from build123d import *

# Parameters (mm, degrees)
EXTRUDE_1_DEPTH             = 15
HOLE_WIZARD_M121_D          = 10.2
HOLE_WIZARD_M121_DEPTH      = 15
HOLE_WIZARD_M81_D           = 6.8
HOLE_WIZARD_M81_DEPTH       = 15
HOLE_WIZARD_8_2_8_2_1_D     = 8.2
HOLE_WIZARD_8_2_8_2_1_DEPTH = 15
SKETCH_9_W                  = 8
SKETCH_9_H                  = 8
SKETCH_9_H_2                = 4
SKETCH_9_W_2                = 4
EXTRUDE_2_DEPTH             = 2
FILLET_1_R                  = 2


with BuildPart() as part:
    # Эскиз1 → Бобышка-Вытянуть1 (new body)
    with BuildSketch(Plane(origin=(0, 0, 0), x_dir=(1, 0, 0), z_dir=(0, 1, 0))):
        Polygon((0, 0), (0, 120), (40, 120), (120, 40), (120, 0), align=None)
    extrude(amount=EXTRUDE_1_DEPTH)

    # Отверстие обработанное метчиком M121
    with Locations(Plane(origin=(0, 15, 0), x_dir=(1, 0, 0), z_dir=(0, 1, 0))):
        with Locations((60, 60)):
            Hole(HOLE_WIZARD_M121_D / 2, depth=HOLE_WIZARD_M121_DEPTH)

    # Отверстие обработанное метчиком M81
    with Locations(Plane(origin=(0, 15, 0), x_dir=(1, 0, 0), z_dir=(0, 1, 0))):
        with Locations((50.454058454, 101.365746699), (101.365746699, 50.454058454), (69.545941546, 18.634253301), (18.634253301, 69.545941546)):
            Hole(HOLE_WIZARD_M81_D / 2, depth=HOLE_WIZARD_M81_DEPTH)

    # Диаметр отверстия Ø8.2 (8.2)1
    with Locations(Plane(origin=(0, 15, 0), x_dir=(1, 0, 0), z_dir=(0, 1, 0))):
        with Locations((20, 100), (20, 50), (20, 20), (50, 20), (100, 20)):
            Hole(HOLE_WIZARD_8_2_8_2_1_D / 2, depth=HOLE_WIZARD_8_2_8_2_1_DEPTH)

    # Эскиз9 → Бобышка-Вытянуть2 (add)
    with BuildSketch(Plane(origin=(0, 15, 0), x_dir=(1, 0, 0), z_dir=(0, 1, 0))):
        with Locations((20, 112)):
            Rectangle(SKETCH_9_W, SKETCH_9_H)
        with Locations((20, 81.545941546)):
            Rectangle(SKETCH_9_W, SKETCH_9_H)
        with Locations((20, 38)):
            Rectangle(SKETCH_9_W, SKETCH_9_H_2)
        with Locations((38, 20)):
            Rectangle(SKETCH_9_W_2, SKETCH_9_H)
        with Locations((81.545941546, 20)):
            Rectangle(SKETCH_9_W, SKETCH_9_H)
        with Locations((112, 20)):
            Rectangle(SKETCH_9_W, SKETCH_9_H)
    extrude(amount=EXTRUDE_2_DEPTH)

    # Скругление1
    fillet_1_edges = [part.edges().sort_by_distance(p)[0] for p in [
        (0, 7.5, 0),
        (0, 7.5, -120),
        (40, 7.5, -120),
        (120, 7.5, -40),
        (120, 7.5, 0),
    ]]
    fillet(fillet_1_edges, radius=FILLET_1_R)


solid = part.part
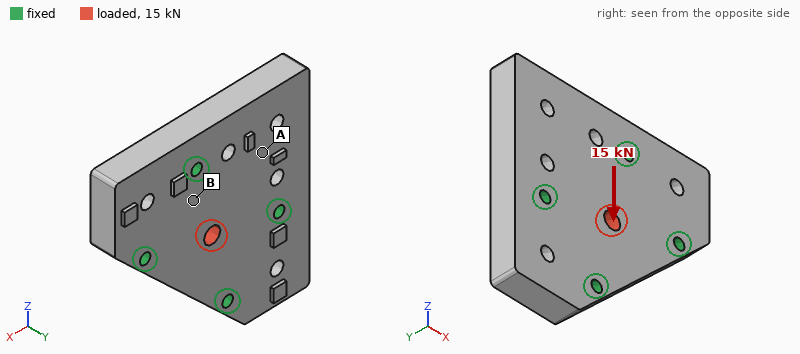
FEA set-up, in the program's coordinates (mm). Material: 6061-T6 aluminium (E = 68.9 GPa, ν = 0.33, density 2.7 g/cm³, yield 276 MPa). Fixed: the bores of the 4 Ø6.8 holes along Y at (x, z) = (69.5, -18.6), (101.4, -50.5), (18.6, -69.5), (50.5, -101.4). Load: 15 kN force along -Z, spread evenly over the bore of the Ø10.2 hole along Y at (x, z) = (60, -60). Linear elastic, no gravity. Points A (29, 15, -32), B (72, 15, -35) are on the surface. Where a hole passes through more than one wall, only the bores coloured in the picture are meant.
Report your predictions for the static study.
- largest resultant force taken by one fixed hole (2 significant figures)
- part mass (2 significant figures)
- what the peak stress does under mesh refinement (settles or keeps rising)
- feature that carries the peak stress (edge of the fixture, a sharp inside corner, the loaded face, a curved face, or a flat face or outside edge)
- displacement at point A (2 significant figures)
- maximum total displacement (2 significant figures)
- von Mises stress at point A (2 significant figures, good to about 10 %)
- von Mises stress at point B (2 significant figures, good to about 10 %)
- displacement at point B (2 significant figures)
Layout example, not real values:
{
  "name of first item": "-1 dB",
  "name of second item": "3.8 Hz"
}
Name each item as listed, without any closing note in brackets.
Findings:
{
  "largest resultant force taken by one fixed hole": "5.6 kN",
  "part mass": "440 g",
  "what the peak stress does under mesh refinement": "keeps rising",
  "feature that carries the peak stress": "a sharp inside corner",
  "displacement at point A": "4.3 µm",
  "maximum total displacement": "12 µm",
  "von Mises stress at point A": "3.5 MPa",
  "von Mises stress at point B": "16 MPa",
  "displacement at point B": "3.4 µm"
}
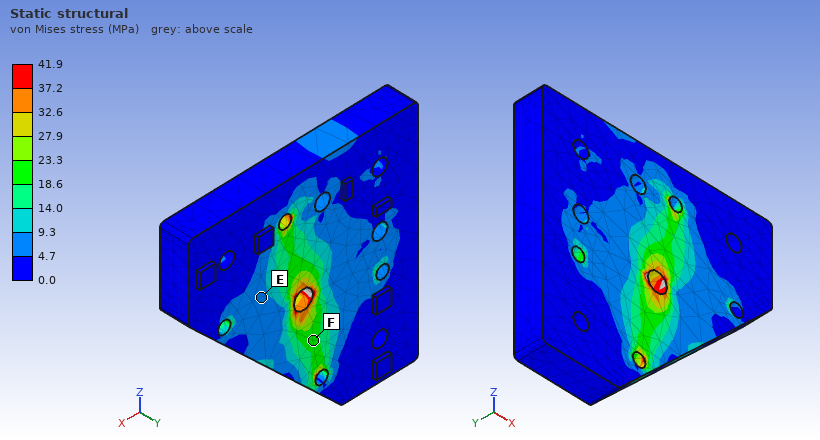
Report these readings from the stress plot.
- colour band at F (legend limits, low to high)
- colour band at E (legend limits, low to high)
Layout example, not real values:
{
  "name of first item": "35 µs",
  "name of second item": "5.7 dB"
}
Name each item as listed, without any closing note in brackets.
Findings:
{
  "colour band at F": "18.6 to 23.3 MPa",
  "colour band at E": "4.7 to 9.3 MPa"
}
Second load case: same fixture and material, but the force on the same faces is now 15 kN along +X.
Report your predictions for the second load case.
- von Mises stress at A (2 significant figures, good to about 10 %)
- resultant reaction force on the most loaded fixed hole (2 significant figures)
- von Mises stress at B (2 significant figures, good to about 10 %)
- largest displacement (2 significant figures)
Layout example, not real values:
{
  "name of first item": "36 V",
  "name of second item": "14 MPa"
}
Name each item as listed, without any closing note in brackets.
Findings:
{
  "von Mises stress at A": "3.3 MPa",
  "resultant reaction force on the most loaded fixed hole": "5.6 kN",
  "von Mises stress at B": "5.8 MPa",
  "largest displacement": "12 µm"
}
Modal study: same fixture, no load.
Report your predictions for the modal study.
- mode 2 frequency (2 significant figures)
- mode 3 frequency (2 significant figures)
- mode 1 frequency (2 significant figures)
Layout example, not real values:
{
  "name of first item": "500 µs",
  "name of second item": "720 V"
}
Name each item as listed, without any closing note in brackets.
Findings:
{
  "mode 2 frequency": "7100 Hz",
  "mode 3 frequency": "7200 Hz",
  "mode 1 frequency": "4200 Hz"
}
